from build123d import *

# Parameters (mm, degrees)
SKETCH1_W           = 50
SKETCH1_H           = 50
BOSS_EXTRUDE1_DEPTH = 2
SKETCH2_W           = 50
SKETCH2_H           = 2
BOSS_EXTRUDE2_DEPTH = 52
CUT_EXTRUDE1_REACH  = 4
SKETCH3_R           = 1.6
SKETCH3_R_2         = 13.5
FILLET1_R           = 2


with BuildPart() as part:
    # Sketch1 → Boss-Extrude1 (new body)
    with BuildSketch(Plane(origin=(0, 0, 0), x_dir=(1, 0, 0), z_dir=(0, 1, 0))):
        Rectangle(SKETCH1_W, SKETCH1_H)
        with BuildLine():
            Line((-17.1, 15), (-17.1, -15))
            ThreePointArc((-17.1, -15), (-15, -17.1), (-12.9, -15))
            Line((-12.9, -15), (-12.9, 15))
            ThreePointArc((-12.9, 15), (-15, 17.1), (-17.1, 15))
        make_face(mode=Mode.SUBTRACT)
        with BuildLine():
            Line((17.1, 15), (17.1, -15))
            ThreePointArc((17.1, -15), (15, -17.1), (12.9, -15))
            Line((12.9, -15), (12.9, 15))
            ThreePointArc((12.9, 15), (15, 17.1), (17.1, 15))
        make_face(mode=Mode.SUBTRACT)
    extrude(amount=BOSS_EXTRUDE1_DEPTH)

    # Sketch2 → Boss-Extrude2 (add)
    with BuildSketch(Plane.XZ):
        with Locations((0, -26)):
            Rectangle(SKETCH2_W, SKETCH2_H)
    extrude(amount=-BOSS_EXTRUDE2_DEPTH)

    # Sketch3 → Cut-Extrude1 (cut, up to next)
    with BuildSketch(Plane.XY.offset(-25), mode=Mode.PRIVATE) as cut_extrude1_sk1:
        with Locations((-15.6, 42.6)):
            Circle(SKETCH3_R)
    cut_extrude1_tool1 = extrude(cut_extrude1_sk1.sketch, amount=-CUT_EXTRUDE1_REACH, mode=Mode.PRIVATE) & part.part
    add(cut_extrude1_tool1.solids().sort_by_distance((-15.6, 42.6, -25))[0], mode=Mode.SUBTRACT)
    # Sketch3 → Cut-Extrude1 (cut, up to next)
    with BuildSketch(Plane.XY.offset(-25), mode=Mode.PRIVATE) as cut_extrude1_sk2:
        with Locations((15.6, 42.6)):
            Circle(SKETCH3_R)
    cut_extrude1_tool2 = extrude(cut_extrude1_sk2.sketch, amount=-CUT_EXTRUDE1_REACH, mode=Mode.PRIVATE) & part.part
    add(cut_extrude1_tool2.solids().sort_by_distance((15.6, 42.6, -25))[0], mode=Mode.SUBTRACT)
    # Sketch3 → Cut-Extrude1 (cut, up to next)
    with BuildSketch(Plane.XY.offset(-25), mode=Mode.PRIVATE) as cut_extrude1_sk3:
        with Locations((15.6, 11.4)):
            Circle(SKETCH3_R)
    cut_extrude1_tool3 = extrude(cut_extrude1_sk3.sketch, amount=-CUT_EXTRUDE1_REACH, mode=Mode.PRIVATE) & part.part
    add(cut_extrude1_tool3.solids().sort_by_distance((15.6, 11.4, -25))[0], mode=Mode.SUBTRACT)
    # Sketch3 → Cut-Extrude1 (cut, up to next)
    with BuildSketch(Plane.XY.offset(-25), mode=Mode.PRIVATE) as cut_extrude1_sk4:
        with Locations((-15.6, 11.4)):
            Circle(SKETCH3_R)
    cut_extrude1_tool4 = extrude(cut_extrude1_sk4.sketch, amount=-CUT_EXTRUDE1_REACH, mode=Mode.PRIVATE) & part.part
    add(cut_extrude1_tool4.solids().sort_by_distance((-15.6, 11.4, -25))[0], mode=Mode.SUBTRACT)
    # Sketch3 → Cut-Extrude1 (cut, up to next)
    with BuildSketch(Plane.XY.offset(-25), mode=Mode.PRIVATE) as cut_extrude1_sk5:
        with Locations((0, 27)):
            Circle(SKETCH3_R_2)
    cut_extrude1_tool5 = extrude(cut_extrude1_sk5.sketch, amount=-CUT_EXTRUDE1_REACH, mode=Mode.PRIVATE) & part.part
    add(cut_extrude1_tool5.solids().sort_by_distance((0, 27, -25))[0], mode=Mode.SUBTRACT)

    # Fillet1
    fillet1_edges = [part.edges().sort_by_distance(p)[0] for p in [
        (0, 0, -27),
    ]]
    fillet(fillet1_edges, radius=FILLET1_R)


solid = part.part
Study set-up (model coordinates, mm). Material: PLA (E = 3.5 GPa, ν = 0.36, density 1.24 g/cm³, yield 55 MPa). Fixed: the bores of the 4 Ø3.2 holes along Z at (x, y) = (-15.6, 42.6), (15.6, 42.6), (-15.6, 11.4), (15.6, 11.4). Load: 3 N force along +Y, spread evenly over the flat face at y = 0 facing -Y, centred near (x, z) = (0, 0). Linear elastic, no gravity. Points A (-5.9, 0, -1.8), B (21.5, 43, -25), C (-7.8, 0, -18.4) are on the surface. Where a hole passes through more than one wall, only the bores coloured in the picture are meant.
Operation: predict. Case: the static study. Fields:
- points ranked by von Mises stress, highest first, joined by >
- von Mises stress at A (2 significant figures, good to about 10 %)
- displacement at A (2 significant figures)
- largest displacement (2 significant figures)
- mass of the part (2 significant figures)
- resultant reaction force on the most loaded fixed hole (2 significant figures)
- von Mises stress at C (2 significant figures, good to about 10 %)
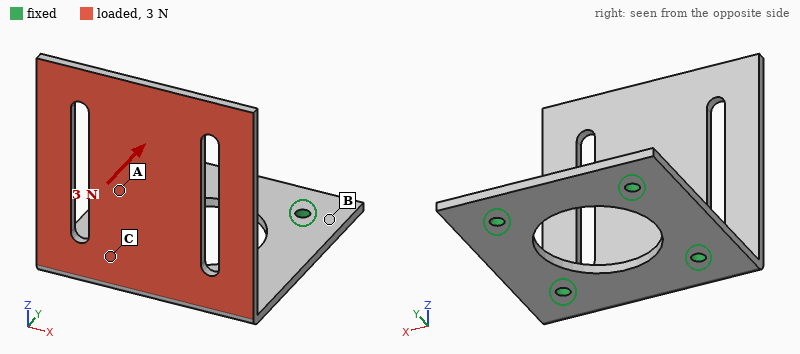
C > A > B
0.77 MPa
0.31 mm
0.80 mm
10 g
1.7 N
1.6 MPa
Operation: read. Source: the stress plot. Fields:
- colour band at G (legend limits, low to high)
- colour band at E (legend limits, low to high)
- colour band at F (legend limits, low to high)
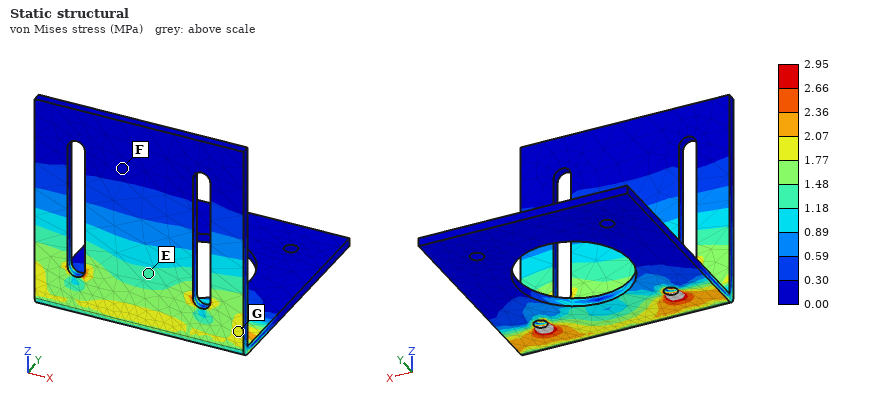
1.77 to 2.07 MPa
1.18 to 1.48 MPa
0.00 to 0.30 MPa
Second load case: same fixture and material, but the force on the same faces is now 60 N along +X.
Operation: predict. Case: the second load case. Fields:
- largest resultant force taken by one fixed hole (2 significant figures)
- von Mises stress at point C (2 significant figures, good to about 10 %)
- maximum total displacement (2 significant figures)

58 N
3.4 MPa
0.92 mm
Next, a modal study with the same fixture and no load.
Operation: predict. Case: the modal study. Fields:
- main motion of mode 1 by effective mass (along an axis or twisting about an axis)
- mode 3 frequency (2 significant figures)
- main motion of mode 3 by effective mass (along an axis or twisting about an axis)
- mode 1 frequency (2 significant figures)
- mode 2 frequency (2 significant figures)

along Y
700 Hz
along X
160 Hz
440 Hz
